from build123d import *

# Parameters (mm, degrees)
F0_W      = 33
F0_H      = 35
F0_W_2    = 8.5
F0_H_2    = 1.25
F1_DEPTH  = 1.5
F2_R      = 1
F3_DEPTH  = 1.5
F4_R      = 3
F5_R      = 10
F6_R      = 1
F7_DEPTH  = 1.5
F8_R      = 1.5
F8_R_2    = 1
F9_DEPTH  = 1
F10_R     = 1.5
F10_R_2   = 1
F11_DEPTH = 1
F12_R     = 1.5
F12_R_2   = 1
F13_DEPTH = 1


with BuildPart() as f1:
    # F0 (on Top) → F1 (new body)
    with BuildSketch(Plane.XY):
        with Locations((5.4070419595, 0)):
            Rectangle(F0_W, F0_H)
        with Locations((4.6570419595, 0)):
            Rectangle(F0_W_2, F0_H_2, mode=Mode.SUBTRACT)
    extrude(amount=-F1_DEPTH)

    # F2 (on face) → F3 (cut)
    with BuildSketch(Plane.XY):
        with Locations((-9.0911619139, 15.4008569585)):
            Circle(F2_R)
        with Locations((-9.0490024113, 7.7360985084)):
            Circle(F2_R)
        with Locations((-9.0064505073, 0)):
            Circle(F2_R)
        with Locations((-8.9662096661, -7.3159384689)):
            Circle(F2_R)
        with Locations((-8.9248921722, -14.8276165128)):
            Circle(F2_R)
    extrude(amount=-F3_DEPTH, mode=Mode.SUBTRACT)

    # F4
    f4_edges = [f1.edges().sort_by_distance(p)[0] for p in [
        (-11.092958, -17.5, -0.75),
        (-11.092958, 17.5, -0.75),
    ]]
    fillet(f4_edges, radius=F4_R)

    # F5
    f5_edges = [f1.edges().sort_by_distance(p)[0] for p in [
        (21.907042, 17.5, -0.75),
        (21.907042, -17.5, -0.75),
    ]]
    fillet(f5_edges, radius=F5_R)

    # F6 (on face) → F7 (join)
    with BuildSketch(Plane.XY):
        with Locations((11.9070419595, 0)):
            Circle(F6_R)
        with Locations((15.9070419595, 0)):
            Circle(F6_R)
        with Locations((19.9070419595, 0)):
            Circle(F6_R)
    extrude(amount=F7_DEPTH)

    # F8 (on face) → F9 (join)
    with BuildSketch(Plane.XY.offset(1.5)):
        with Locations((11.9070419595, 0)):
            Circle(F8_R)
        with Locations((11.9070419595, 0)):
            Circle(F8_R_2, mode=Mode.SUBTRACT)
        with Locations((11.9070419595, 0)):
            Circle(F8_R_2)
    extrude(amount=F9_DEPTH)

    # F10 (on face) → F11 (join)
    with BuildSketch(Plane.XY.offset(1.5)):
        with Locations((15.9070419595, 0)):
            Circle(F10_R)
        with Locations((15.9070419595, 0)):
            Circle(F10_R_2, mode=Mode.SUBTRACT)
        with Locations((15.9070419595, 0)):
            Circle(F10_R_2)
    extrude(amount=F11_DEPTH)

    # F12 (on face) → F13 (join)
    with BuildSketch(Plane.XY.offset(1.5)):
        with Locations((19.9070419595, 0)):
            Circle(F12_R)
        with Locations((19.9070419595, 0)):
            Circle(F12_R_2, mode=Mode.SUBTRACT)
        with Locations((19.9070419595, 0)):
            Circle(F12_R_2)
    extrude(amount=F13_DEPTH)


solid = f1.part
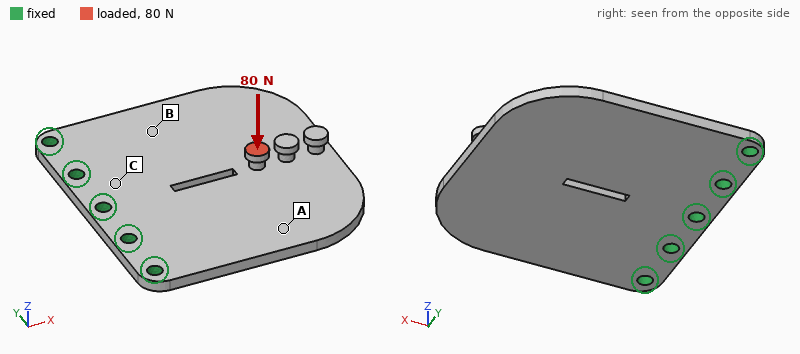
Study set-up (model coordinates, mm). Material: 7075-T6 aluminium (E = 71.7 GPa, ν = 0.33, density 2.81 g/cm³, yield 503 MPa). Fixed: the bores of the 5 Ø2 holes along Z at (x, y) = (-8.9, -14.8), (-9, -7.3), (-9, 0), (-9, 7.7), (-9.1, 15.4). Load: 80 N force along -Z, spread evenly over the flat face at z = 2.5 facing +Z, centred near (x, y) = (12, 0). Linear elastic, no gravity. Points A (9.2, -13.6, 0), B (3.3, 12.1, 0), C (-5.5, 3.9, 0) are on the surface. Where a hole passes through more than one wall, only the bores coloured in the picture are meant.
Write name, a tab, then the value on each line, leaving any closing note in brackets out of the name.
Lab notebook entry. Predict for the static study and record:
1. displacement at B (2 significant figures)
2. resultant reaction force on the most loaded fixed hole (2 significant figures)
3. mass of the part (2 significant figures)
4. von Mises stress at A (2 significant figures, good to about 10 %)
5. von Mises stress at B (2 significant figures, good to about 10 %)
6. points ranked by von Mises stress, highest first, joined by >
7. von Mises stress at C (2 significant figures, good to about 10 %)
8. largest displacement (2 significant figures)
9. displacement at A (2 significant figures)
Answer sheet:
displacement at B	0.12 mm
resultant reaction force on the most loaded fixed hole	30 N
mass of the part	4.7 g
von Mises stress at A	26 MPa
von Mises stress at B	53 MPa
points ranked by von Mises stress, highest first, joined by >	C > B > A
von Mises stress at C	99 MPa
largest displacement	0.57 mm
displacement at A	0.24 mm
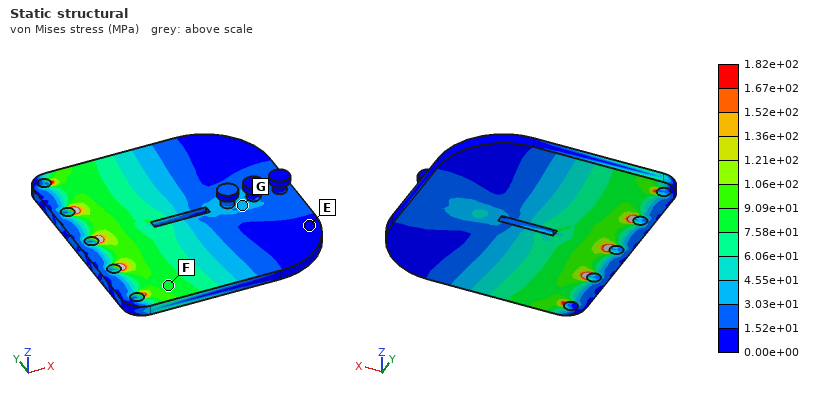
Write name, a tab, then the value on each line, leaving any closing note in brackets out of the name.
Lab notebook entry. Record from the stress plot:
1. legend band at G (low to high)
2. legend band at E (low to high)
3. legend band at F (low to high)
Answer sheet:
legend band at G	3.03e+01 to 4.55e+01 MPa
legend band at E	0.00e+00 to 1.52e+01 MPa
legend band at F	7.58e+01 to 9.09e+01 MPa
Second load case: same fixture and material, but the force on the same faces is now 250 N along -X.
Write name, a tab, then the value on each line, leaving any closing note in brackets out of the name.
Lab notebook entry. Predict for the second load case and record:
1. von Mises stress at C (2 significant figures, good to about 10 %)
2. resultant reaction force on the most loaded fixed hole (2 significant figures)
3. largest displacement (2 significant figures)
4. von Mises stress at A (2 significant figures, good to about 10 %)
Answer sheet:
von Mises stress at C	57 MPa
resultant reaction force on the most loaded fixed hole	54 N
largest displacement	0.49 mm
von Mises stress at A	45 MPa
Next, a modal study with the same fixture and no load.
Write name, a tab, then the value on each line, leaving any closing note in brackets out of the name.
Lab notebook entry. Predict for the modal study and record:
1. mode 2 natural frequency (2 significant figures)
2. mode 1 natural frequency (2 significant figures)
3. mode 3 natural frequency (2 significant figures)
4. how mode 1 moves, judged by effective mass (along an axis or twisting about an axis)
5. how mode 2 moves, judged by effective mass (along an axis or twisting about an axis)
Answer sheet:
mode 2 natural frequency	3300 Hz
mode 1 natural frequency	1400 Hz
mode 3 natural frequency	7700 Hz
how mode 1 moves, judged by effective mass	along Z
how mode 2 moves, judged by effective mass	twisting about X
